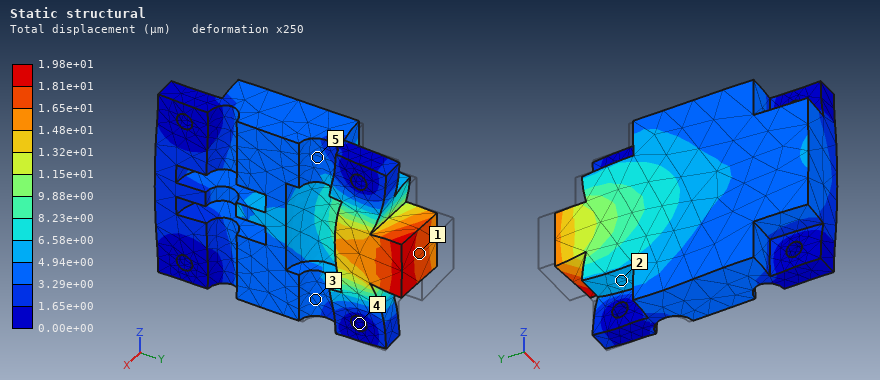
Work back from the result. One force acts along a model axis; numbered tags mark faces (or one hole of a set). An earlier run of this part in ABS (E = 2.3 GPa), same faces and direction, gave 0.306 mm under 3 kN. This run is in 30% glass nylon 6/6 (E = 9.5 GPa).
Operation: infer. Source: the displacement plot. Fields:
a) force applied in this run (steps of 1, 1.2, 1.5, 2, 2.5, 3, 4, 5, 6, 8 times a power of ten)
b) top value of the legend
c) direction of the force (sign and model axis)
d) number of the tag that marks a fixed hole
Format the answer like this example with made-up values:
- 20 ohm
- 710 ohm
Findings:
- 800 N
- 1.98e+01 µm
- -Y
- 4
